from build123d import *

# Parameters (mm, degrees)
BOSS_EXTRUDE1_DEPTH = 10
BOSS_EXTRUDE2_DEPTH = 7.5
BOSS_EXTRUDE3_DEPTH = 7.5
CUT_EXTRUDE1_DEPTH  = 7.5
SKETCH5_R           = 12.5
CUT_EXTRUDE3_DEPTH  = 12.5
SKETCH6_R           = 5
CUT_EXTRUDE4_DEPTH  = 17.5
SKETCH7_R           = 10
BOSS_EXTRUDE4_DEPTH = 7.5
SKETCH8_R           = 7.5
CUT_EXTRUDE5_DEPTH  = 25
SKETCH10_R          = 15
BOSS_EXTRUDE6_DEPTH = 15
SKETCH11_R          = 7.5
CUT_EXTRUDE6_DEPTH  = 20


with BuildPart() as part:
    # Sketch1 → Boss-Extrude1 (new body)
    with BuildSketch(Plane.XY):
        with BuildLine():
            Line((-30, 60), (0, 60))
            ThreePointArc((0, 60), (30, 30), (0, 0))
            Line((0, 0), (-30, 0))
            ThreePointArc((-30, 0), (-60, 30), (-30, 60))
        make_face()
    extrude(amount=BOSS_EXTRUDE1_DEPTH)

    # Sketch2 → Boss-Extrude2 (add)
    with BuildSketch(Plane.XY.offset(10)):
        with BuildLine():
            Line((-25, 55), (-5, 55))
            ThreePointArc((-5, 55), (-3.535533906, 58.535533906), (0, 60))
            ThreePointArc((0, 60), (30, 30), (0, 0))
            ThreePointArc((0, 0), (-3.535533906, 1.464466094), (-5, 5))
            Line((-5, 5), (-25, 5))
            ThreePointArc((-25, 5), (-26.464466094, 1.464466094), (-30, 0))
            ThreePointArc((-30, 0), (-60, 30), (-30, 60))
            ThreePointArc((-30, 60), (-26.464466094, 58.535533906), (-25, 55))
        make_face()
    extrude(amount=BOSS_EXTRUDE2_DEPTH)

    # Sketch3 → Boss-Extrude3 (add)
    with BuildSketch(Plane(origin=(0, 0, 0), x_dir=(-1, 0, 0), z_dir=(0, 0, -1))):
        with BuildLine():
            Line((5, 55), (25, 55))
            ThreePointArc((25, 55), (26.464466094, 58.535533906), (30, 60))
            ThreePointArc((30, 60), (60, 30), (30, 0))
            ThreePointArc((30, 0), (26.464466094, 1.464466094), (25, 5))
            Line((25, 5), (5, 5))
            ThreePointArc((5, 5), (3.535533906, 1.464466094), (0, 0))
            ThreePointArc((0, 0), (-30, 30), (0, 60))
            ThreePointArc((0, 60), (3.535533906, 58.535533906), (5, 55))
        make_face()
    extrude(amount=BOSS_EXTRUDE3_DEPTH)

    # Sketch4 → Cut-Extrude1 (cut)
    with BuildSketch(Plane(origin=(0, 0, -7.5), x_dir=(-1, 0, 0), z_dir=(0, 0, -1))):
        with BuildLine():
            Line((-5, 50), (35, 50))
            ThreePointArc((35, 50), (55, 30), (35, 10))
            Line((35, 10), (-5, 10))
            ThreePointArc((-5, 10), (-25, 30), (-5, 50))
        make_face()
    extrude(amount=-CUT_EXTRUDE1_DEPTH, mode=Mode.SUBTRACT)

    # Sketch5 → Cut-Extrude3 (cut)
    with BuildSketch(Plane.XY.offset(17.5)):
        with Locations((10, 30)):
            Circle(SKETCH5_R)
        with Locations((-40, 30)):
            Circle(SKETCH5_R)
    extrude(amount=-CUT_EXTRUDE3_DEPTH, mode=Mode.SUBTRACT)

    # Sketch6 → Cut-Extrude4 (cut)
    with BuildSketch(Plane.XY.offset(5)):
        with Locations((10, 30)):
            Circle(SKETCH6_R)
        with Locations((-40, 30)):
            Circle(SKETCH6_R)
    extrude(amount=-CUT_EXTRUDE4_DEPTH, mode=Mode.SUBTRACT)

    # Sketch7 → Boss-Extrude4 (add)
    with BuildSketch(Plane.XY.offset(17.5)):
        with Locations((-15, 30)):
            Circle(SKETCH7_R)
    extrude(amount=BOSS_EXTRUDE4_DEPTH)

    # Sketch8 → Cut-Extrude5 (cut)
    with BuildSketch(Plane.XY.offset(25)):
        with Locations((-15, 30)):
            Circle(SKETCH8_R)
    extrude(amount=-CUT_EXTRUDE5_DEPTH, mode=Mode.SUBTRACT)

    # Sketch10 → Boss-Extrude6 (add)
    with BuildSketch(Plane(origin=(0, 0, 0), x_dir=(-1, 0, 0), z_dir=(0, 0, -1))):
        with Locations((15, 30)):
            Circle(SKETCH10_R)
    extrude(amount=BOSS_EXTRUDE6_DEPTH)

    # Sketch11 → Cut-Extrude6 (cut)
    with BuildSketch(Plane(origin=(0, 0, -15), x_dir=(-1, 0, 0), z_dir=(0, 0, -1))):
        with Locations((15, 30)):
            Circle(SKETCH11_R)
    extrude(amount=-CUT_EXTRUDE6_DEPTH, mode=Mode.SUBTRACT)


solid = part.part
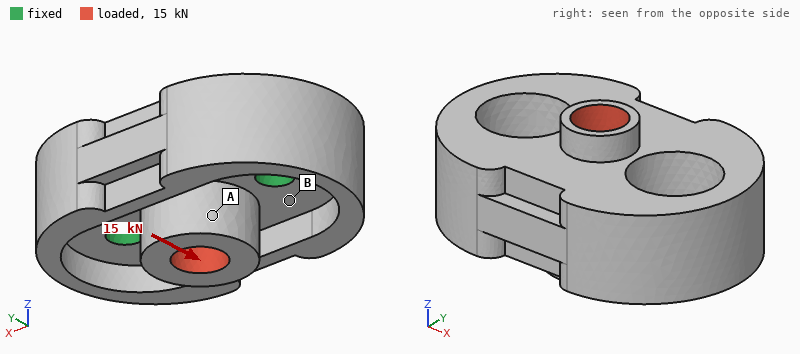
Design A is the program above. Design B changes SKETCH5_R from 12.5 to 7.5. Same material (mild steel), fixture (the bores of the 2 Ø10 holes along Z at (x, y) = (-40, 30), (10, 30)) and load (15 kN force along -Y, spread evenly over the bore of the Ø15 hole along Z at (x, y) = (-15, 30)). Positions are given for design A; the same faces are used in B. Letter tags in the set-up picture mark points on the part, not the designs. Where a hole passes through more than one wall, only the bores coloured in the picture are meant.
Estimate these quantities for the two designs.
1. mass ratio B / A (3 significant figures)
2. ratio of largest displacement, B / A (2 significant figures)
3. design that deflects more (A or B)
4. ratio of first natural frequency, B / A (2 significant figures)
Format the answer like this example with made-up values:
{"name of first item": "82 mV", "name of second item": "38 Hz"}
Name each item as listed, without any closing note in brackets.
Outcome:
{"mass ratio B / A": "1.09", "ratio of largest displacement, B / A": "0.76", "design that deflects more": "A", "ratio of first natural frequency, B / A": "1.2"}
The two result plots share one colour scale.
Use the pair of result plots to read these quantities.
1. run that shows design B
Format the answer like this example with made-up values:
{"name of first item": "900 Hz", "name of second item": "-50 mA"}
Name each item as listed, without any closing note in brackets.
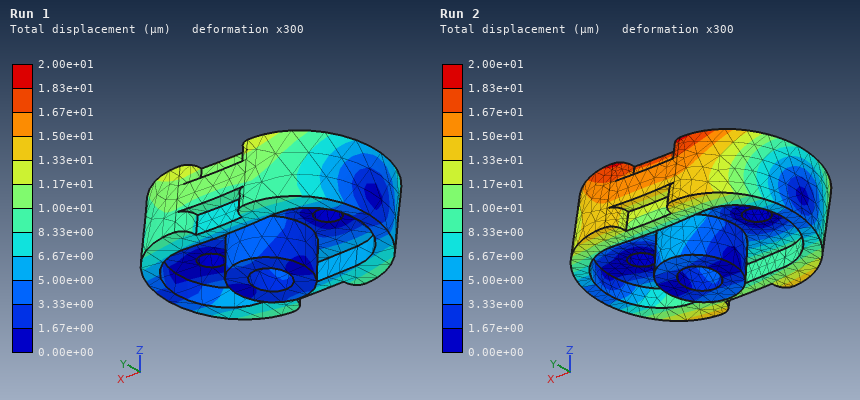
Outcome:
{"run that shows design B": "Run 1"}
